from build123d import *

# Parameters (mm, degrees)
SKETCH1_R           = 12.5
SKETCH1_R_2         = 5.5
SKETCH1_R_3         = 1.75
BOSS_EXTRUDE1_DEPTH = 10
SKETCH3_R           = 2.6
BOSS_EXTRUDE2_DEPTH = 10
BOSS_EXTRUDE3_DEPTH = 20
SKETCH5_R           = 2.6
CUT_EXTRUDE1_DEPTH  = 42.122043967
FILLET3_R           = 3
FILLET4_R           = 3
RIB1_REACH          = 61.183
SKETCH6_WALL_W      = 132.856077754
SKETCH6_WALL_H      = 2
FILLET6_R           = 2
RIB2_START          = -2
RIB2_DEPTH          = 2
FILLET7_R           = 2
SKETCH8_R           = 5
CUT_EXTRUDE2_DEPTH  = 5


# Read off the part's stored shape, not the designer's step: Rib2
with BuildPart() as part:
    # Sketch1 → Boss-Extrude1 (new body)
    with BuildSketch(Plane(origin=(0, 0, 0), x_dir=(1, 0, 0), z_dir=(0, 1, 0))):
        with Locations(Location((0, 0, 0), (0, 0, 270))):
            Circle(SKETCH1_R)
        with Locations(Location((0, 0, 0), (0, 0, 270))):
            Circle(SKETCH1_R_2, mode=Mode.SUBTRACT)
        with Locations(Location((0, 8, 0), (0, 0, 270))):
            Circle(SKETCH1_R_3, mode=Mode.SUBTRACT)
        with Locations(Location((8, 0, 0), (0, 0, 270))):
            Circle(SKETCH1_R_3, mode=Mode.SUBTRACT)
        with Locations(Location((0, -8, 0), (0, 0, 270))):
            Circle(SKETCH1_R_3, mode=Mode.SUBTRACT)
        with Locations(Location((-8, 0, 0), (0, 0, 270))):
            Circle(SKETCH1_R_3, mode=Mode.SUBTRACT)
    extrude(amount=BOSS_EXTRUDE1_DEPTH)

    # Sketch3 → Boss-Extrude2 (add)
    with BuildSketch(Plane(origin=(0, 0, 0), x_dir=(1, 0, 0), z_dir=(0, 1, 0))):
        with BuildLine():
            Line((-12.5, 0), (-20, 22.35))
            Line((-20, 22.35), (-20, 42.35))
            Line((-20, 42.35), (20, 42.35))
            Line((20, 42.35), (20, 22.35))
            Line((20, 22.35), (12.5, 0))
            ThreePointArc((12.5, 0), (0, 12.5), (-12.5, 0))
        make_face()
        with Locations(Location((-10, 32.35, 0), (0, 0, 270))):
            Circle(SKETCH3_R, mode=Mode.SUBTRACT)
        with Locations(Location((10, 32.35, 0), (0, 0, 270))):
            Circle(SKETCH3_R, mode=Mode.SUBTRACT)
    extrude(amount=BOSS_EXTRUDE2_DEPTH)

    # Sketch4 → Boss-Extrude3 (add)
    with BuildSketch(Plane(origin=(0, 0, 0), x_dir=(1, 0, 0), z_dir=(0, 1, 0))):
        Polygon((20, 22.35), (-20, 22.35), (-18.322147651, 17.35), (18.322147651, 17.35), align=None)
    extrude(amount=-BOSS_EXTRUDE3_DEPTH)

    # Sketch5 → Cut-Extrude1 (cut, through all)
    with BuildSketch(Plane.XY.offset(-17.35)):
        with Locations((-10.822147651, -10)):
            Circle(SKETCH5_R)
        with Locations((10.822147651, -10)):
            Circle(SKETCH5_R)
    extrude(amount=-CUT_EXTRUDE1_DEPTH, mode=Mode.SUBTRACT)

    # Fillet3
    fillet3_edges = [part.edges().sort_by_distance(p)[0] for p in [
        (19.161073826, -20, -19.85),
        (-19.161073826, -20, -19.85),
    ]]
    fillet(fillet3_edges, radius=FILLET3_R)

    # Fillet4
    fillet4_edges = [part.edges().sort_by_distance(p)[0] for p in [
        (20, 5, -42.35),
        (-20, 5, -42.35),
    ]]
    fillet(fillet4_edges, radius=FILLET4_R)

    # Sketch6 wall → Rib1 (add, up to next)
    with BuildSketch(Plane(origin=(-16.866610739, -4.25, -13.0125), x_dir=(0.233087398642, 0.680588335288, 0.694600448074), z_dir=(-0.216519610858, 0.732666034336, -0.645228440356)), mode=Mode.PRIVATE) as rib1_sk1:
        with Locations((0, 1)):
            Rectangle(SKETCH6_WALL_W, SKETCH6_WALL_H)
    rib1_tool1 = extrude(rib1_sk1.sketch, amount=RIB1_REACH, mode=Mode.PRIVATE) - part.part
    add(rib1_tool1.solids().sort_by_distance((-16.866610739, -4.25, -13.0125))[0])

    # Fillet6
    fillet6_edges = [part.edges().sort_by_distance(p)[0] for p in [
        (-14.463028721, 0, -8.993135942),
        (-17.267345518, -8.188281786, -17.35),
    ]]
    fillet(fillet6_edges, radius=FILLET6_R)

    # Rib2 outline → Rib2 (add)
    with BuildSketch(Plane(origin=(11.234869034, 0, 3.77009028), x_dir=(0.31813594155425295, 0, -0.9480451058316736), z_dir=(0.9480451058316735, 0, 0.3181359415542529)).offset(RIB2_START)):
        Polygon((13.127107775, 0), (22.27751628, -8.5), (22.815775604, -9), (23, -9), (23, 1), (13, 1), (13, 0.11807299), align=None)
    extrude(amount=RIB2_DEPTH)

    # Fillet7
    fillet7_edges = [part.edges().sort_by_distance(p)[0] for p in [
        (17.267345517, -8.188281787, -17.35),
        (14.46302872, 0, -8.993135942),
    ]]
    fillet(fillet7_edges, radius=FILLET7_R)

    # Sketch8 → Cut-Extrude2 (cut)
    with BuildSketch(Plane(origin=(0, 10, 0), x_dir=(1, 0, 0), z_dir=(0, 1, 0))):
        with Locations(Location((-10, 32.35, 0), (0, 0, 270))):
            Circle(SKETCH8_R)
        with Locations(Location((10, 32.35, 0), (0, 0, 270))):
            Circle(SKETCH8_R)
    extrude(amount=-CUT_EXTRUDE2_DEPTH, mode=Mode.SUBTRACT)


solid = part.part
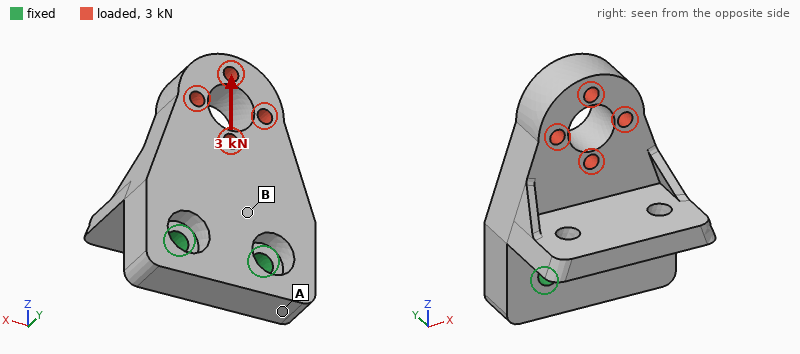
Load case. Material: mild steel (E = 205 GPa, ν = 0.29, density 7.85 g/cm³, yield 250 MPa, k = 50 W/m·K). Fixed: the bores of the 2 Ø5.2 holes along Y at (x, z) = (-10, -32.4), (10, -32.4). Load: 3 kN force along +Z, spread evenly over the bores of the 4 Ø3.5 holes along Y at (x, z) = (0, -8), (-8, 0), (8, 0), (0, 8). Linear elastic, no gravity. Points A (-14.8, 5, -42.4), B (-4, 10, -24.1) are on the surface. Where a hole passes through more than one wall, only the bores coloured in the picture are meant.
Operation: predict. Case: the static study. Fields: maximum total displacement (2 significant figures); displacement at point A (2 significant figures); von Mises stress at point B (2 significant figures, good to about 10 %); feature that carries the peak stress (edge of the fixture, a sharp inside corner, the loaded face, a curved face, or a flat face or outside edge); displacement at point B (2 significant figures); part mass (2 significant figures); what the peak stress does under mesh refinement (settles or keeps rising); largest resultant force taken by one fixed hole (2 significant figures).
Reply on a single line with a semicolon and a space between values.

11 µm; 1.6 µm; 12 MPa; edge of the fixture; 2.6 µm; 150 g; keeps rising; 1.5 kN
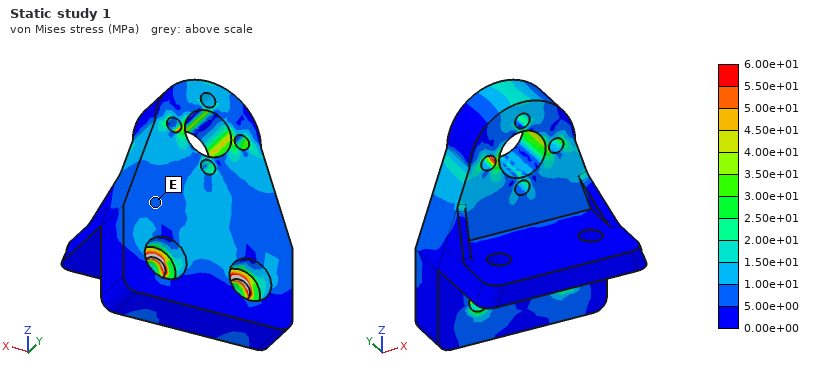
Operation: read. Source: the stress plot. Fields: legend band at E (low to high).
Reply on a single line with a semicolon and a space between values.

5.00e+00 to 1.00e+01 MPa
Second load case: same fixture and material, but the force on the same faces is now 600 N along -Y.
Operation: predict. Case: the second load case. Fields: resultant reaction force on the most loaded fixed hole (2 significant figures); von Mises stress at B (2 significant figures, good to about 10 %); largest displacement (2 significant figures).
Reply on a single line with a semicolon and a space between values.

310 N; 26 MPa; 36 µm
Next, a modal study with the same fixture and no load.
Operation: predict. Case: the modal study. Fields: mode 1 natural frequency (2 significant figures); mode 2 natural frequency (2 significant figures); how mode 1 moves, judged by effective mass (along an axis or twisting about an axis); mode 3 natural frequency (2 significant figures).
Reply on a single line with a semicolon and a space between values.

3600 Hz; 9700 Hz; along Y; 10000 Hz
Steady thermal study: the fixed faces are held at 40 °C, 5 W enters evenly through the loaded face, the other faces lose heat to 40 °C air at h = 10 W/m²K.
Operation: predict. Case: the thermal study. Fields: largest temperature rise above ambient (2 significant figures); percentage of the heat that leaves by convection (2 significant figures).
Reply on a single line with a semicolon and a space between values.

14 K; 7.0 %
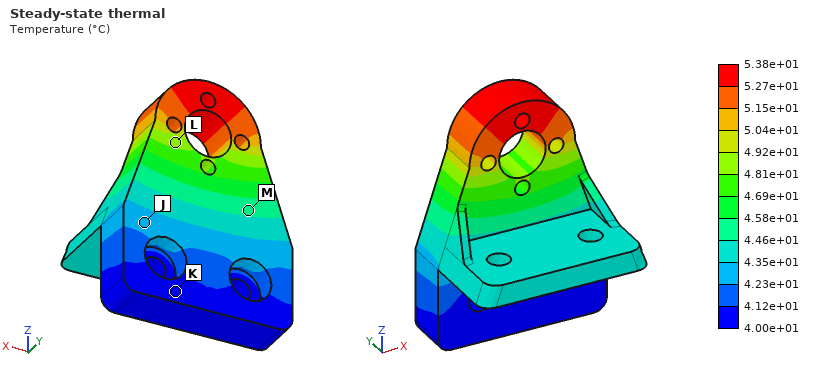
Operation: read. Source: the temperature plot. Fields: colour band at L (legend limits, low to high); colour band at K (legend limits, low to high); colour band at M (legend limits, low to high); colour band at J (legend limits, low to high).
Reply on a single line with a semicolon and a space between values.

4.81e+01 to 4.92e+01 °C; 4.00e+01 to 4.12e+01 °C; 4.46e+01 to 4.58e+01 °C; 4.23e+01 to 4.35e+01 °C
